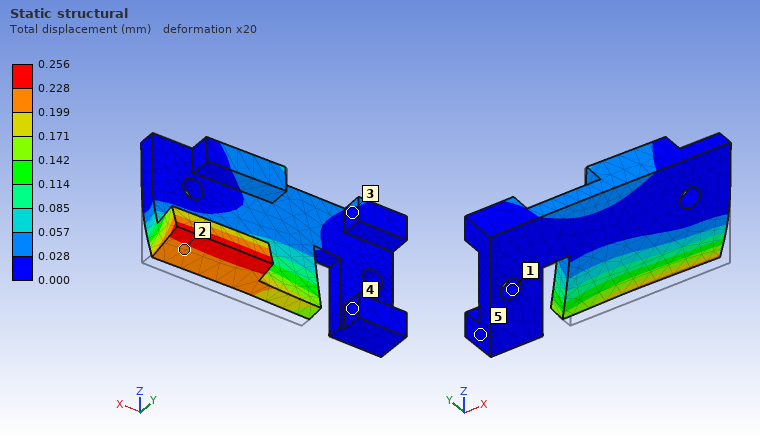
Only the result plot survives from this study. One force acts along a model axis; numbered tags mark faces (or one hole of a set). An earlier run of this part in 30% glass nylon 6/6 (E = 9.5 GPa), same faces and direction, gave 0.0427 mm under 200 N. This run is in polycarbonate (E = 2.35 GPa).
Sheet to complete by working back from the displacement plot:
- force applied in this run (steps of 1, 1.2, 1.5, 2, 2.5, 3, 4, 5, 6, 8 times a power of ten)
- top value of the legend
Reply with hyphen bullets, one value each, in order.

- 300 N
- 0.256 mm
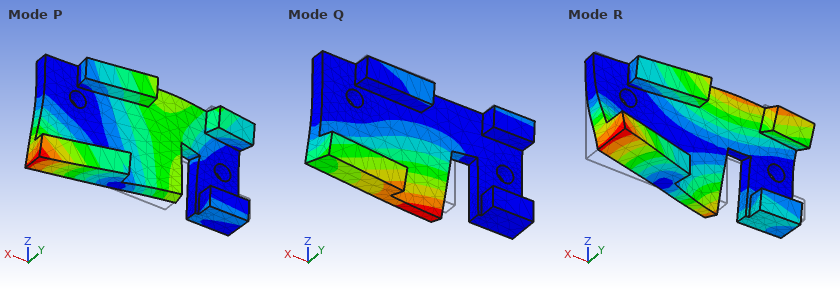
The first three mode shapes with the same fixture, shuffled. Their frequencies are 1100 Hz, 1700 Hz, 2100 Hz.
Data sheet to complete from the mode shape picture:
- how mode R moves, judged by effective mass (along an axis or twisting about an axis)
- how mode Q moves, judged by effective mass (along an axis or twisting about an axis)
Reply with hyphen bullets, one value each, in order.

- along Y
- along Y
